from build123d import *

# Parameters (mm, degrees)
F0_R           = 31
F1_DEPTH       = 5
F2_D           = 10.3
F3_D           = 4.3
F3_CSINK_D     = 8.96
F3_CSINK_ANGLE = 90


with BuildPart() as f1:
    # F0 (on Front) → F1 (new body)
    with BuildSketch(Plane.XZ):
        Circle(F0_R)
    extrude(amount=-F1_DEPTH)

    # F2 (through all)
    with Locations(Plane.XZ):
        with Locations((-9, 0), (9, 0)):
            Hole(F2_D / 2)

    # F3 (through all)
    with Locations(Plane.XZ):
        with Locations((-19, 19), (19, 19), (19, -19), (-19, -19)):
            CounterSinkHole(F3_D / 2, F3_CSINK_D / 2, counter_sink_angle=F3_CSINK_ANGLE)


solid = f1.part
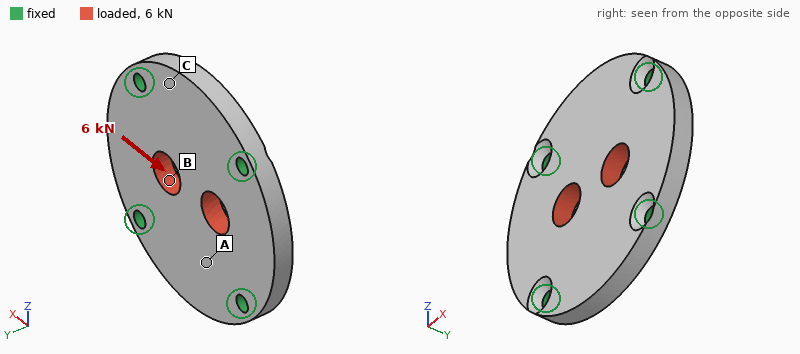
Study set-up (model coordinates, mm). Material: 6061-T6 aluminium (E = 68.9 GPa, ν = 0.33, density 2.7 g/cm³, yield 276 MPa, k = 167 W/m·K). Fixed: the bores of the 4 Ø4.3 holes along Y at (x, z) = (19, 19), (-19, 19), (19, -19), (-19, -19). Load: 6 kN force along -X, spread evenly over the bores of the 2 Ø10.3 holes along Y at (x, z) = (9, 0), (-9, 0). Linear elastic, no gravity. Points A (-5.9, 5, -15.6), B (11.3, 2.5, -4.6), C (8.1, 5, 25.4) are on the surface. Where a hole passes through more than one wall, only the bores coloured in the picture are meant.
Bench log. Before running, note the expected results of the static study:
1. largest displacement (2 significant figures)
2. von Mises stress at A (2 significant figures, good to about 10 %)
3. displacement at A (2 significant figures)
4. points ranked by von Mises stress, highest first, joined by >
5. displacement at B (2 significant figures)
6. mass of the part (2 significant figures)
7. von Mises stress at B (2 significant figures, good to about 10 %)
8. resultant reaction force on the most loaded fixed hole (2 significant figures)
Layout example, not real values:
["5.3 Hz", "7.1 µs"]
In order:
["13 µm", "17 MPa", "4.6 µm", "B > A > C", "9.3 µm", "37 g", "30 MPa", "1.5 kN"]
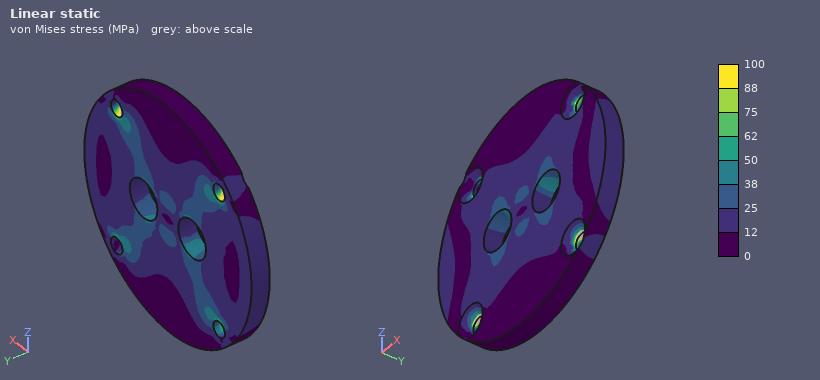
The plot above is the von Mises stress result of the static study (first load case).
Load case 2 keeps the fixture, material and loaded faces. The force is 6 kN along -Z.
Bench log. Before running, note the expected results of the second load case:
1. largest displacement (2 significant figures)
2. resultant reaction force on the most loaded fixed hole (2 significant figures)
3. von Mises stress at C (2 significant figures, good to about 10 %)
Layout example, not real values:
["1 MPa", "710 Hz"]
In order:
["10 µm", "1.5 kN", "10 MPa"]
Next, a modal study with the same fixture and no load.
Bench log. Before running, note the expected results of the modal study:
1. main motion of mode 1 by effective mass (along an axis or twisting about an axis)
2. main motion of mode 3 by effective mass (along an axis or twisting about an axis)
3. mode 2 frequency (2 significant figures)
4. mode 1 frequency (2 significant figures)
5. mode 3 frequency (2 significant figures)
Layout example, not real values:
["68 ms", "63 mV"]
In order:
["along Y", "twisting about X", "11 kHz", "11 kHz", "12 kHz"]
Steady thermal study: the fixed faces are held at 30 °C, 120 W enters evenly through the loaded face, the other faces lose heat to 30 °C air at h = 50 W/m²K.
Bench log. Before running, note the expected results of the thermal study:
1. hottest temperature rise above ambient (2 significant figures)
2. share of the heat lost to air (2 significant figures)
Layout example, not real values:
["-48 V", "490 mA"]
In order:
["43 K", "4.5 %"]
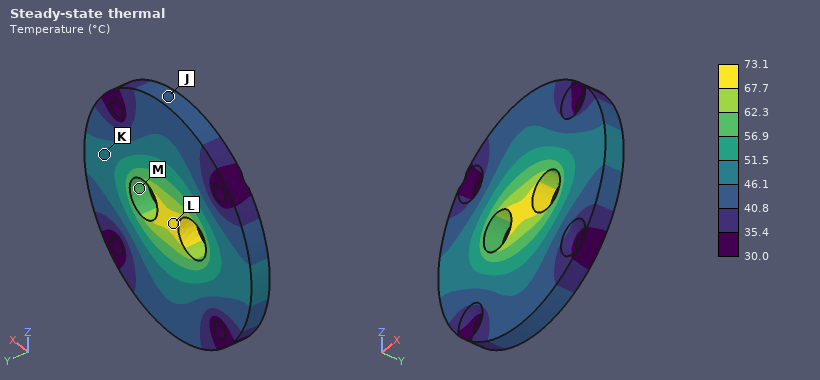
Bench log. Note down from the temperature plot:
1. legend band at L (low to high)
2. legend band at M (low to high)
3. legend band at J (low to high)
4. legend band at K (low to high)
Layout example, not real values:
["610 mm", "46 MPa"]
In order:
["67.7 to 73.1 °C", "56.9 to 62.3 °C", "40.8 to 46.1 °C", "46.1 to 51.5 °C"]
